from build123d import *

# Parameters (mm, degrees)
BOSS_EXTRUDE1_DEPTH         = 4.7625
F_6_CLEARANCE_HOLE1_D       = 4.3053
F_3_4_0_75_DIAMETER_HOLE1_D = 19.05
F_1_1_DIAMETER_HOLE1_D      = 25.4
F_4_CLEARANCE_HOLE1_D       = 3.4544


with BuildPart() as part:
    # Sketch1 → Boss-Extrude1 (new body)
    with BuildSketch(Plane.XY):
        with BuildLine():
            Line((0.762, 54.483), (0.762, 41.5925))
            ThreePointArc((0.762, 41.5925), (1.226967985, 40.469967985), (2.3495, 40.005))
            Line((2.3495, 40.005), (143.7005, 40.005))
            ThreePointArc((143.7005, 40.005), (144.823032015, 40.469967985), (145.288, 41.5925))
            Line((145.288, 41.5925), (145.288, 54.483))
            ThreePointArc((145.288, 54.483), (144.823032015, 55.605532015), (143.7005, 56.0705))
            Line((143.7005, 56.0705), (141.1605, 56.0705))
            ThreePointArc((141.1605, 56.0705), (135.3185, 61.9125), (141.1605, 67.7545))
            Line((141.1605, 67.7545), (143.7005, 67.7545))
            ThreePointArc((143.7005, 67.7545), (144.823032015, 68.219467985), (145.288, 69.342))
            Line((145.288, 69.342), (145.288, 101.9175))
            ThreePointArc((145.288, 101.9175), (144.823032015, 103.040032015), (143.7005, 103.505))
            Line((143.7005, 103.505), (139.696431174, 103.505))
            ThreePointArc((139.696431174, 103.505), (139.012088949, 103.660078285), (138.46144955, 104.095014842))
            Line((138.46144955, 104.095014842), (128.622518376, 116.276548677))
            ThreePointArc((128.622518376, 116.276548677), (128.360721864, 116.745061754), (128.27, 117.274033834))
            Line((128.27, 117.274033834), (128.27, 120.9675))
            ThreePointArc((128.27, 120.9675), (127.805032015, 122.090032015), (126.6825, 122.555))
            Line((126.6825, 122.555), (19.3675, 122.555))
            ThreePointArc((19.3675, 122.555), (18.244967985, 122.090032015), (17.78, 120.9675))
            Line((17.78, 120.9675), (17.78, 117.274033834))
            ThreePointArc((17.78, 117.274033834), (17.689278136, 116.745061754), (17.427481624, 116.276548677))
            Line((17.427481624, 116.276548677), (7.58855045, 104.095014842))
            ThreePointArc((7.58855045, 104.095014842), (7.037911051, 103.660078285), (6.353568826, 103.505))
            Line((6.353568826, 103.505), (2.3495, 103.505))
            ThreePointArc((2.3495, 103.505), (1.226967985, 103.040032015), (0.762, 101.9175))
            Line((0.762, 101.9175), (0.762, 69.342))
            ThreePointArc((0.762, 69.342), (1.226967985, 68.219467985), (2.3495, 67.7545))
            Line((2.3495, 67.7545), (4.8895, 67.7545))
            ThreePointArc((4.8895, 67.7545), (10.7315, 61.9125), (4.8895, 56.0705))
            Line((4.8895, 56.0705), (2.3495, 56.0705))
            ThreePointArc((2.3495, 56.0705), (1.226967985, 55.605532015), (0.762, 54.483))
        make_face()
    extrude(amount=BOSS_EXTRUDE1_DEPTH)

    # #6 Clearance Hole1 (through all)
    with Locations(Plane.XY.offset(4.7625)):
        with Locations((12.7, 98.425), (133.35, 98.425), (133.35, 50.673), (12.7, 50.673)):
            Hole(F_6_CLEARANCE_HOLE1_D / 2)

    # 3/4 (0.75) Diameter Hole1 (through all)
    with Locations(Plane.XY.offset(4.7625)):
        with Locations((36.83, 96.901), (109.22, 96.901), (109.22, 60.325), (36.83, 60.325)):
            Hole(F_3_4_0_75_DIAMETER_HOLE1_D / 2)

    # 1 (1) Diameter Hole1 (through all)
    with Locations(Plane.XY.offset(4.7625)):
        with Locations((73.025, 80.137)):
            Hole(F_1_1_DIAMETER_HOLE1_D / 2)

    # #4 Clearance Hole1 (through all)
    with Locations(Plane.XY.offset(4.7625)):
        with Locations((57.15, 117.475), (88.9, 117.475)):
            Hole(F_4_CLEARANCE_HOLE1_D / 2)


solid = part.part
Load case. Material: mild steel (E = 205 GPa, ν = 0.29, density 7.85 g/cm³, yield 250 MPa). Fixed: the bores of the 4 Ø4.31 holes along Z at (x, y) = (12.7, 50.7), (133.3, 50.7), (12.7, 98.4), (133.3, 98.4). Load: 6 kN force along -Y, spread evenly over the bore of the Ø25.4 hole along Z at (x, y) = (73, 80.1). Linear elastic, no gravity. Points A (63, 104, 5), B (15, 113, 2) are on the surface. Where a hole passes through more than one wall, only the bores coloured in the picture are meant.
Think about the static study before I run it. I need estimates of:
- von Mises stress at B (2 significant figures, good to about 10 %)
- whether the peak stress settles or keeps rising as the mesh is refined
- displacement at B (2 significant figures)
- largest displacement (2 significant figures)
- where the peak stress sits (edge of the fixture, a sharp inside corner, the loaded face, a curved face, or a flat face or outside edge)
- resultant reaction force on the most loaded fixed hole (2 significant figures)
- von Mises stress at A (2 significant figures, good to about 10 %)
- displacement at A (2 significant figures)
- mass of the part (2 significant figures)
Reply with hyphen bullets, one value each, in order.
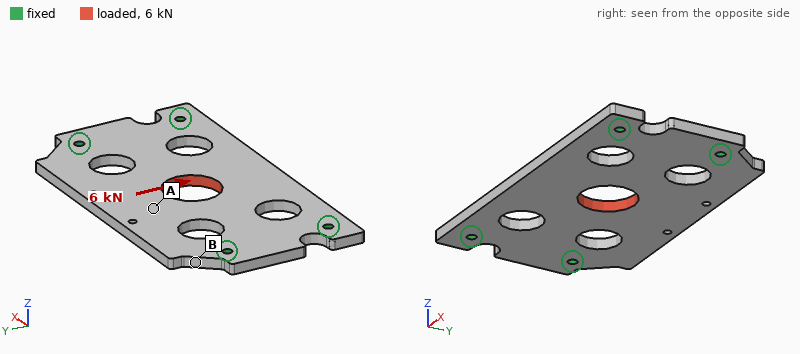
- 6.4 MPa
- keeps rising
- 2.4 µm
- 14 µm
- edge of the fixture
- 1.9 kN
- 13 MPa
- 13 µm
- 350 g
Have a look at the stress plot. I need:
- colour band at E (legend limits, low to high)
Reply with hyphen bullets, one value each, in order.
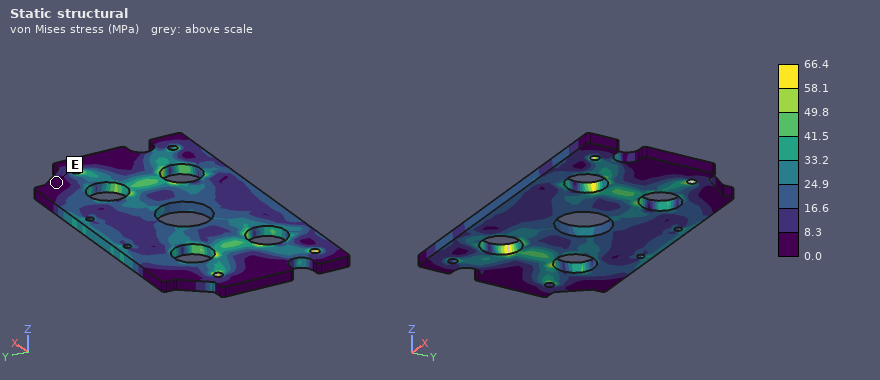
- 0.0 to 8.3 MPa
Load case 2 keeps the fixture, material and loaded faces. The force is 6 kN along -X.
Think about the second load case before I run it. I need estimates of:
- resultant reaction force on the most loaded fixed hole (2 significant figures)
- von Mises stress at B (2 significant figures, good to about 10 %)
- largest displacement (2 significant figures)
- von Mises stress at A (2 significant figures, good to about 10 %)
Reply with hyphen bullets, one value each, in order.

- 1.7 kN
- 7.6 MPa
- 6.0 µm
- 7.5 MPa
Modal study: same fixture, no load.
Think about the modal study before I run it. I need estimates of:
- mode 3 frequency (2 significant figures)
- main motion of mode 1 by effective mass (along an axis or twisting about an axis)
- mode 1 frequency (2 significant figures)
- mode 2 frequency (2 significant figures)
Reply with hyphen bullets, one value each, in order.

- 3900 Hz
- along Z
- 1500 Hz
- 2000 Hz
